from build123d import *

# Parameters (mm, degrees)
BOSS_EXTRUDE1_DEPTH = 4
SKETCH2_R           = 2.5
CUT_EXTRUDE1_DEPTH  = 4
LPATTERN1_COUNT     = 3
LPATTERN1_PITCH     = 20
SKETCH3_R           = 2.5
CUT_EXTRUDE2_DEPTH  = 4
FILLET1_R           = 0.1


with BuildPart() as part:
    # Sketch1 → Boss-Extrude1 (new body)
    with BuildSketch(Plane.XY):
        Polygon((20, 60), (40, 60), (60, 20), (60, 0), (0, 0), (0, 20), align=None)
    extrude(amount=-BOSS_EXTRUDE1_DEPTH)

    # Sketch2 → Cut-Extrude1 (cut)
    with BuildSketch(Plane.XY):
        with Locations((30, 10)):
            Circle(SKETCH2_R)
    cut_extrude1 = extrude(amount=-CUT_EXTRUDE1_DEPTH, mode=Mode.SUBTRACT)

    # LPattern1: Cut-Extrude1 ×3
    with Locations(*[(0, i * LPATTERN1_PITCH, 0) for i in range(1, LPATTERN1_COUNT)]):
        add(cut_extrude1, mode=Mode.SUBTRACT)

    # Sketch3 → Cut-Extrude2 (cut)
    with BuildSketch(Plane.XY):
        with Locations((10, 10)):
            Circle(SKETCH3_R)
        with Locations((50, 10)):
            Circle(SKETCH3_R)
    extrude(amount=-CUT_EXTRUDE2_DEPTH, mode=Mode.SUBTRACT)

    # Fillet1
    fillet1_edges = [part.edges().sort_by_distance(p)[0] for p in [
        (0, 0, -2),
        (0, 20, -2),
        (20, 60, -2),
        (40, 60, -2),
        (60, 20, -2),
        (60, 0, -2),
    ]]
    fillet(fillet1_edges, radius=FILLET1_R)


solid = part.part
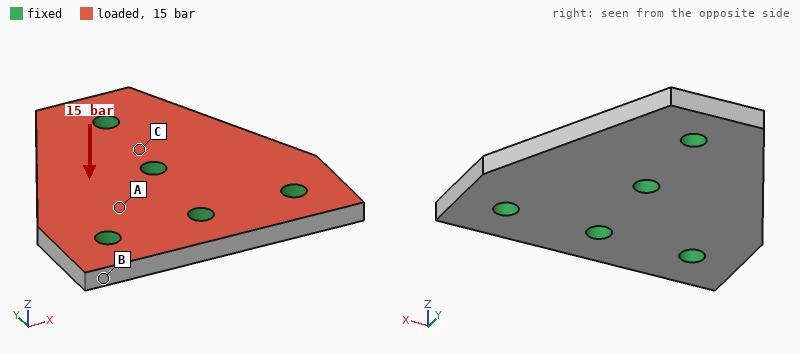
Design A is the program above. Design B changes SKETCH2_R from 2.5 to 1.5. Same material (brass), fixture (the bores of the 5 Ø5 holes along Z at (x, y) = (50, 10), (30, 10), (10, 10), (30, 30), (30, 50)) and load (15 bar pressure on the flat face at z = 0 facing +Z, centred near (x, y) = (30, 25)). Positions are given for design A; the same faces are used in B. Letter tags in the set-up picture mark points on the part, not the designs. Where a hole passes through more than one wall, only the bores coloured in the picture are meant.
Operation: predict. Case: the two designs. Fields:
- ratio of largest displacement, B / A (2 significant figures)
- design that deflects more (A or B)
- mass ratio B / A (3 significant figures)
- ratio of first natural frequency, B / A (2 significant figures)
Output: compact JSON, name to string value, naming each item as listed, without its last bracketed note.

{"ratio of largest displacement, B / A": "1.1", "design that deflects more": "B", "mass ratio B / A": "1.01", "ratio of first natural frequency, B / A": "0.88"}
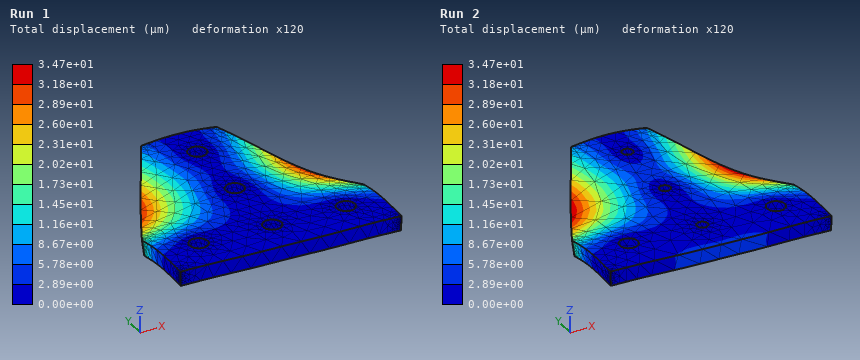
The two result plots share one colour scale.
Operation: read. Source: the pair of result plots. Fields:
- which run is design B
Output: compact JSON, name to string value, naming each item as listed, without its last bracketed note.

{"which run is design B": "Run 2"}
